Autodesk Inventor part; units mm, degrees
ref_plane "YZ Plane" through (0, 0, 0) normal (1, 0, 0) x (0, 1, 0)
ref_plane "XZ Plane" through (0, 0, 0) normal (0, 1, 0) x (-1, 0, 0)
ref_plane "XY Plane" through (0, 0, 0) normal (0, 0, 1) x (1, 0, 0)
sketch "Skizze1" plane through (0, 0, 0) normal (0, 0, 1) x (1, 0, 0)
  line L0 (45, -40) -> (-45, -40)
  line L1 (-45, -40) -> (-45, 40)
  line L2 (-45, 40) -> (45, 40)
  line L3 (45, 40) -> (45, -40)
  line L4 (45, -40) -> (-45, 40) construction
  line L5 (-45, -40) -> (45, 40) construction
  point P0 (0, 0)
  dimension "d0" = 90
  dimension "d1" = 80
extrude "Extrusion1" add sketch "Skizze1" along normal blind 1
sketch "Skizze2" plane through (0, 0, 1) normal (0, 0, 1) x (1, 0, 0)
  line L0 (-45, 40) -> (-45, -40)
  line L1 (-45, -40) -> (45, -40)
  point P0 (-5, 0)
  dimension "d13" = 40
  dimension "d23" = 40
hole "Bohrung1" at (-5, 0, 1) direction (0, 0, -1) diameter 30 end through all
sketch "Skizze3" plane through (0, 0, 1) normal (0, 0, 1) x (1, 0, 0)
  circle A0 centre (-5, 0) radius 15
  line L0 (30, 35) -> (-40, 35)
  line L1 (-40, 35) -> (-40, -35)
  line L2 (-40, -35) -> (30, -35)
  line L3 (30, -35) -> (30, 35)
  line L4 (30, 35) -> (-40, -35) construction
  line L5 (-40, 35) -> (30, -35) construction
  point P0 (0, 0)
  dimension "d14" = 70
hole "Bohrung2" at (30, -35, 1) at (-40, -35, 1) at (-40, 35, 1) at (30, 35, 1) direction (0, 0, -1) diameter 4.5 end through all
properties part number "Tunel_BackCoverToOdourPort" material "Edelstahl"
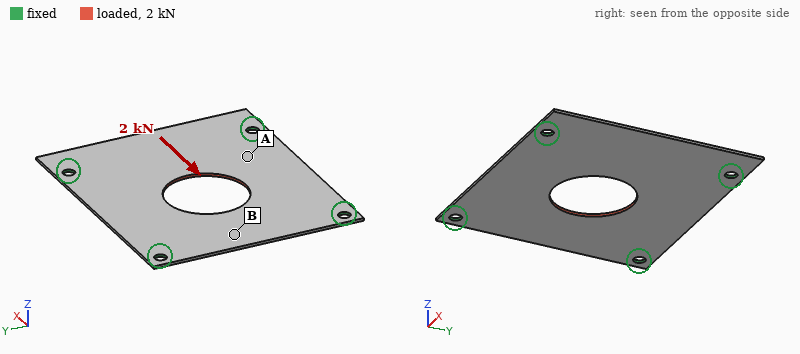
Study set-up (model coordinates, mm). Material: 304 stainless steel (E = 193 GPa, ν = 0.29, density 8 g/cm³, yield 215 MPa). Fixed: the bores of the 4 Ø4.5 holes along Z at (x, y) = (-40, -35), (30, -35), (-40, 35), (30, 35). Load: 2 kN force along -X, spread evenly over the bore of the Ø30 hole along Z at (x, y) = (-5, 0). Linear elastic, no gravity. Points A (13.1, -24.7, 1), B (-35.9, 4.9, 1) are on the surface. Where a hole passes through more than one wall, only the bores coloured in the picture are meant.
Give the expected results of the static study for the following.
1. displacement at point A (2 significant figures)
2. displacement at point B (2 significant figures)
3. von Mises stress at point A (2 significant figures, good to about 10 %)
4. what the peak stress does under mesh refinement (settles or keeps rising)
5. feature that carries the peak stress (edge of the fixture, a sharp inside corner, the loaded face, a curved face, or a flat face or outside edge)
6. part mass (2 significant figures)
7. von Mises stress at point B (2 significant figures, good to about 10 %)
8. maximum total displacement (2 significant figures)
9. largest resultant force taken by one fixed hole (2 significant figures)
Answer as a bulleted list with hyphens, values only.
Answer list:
- 3.5 µm
- 7.0 µm
- 23 MPa
- keeps rising
- edge of the fixture
- 51 g
- 10 MPa
- 8.2 µm
- 550 N
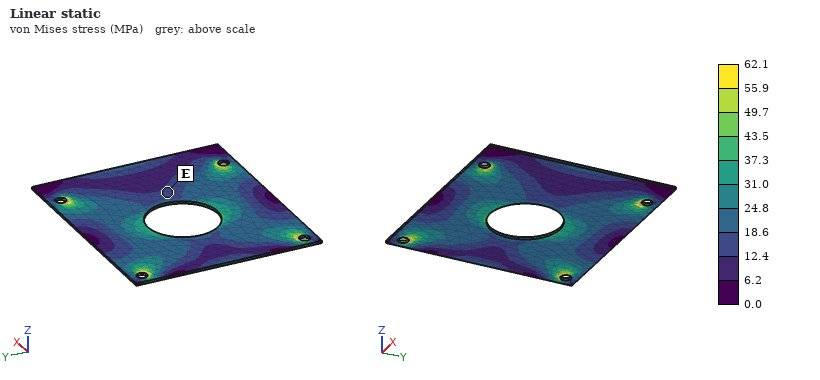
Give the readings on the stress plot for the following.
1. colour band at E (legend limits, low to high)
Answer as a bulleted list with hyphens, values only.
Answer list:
- 12.4 to 18.6 MPa
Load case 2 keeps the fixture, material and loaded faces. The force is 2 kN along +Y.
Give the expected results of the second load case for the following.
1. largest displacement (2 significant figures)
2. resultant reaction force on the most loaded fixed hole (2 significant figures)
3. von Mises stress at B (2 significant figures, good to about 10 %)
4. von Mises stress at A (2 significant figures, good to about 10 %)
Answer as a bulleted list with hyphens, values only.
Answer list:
- 8.1 µm
- 570 N
- 17 MPa
- 25 MPa
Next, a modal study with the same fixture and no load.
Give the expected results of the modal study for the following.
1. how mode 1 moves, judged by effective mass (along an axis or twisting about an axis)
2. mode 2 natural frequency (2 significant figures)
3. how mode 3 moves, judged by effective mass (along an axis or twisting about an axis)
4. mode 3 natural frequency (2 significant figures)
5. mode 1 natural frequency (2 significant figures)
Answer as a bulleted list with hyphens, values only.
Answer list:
- along Z
- 1100 Hz
- twisting about X
- 1200 Hz
- 760 Hz
